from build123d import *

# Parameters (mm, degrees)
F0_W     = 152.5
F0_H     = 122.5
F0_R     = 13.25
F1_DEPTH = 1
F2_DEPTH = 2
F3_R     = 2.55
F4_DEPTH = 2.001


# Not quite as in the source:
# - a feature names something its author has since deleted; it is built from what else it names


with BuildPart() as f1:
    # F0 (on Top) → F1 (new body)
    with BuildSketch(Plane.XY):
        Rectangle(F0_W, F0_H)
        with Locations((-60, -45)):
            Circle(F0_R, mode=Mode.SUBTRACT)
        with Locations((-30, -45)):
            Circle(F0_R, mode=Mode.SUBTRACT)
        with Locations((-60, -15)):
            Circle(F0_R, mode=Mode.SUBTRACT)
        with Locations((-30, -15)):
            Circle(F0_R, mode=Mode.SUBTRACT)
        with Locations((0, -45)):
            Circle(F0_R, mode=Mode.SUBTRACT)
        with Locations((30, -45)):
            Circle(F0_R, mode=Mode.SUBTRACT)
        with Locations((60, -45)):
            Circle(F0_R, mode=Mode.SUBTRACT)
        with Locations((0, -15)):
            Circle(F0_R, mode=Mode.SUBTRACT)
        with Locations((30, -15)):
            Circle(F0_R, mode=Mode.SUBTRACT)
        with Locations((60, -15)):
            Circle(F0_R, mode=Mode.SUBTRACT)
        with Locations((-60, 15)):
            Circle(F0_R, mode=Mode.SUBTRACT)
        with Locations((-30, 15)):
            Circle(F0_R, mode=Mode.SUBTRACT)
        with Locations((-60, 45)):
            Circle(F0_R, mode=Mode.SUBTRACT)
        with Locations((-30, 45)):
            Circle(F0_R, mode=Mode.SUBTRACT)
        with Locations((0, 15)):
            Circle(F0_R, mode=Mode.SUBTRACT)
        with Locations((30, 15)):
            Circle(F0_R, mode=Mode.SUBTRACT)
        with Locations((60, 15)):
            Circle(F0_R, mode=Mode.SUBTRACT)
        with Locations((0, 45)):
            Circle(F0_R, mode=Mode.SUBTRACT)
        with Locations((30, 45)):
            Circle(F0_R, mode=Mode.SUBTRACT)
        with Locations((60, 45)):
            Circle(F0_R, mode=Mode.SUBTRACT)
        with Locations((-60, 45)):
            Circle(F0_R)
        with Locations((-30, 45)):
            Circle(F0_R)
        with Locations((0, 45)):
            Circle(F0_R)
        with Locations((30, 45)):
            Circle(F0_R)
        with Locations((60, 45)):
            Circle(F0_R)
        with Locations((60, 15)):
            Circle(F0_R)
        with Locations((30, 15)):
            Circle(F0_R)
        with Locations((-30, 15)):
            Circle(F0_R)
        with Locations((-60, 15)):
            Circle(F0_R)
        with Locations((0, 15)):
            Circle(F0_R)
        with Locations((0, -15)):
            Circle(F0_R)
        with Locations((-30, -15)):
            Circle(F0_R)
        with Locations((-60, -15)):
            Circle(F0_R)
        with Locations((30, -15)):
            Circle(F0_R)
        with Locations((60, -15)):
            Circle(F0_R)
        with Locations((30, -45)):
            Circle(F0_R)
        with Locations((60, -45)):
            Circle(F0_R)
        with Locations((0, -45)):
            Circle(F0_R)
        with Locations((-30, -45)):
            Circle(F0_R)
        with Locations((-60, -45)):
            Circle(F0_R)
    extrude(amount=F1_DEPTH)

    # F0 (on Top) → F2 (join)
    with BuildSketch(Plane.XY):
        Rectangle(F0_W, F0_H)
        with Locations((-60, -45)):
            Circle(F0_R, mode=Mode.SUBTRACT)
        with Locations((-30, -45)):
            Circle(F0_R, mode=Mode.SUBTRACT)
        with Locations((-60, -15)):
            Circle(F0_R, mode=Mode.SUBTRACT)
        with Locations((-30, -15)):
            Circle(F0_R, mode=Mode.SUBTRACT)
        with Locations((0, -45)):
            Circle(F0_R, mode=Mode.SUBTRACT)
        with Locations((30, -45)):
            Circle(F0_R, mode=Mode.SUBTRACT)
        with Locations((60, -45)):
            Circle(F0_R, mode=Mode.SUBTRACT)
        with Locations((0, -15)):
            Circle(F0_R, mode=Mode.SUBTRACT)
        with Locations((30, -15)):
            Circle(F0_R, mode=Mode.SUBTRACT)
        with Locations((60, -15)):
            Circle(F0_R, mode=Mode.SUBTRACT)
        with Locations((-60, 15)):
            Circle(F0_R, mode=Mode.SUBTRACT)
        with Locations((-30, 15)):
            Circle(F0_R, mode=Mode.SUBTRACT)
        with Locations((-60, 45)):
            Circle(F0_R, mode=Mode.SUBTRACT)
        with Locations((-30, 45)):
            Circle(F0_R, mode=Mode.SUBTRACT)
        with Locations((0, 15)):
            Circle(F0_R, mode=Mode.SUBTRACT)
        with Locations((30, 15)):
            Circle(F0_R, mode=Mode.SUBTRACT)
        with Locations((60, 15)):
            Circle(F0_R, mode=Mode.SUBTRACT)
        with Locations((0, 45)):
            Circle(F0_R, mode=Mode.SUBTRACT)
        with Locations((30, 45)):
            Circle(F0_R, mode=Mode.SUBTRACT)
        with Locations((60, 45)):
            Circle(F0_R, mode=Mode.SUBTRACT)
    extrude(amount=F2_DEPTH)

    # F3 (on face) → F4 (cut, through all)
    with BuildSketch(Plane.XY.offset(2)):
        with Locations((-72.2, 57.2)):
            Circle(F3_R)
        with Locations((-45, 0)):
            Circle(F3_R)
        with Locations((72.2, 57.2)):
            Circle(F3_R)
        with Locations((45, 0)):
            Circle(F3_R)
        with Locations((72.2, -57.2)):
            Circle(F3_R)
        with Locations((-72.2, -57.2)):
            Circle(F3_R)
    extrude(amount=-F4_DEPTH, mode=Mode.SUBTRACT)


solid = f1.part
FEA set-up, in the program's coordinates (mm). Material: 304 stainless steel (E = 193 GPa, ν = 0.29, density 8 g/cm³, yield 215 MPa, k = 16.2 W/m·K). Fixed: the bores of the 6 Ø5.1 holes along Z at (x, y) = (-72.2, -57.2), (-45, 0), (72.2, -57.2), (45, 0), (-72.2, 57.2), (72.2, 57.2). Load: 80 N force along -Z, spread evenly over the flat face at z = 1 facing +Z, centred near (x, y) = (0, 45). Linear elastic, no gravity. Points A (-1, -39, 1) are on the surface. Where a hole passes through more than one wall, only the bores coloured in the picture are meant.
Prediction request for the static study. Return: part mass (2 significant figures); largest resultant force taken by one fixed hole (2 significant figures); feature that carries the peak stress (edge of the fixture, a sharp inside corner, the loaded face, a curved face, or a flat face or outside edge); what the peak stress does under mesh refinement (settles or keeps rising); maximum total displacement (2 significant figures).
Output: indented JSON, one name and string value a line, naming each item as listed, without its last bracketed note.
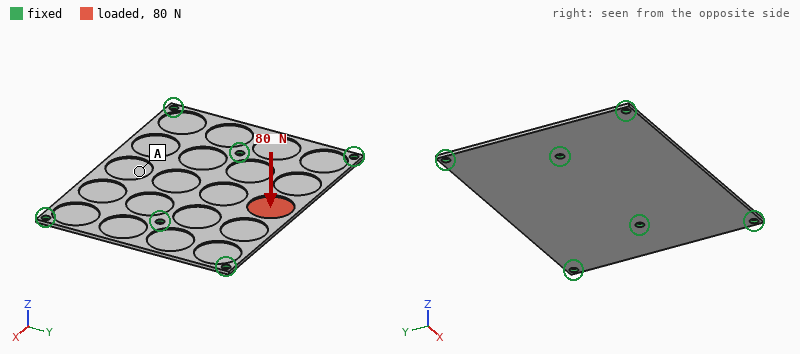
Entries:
{
  "part mass": "210 g",
  "largest resultant force taken by one fixed hole": "44 N",
  "feature that carries the peak stress": "a sharp inside corner",
  "what the peak stress does under mesh refinement": "keeps rising",
  "maximum total displacement": "0.37 mm"
}
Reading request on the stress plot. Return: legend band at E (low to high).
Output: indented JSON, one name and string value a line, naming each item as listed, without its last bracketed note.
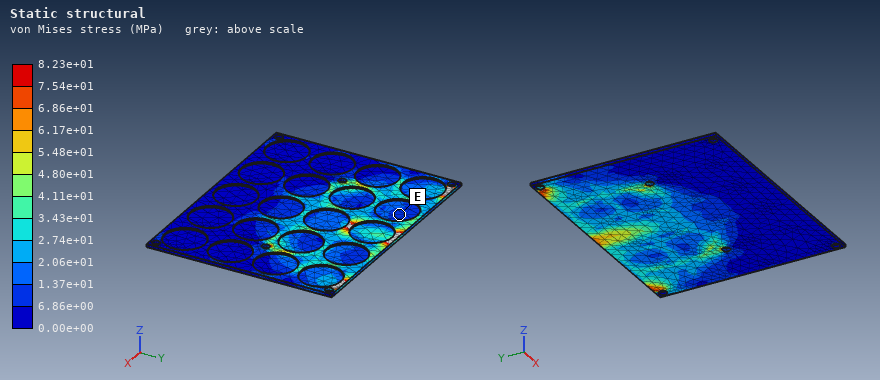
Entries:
{
  "legend band at E": "6.86e+00 to 1.37e+01 MPa"
}
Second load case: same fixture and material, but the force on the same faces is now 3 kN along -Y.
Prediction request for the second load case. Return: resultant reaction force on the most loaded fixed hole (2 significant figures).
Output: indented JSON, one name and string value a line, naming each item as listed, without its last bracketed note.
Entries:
{
  "resultant reaction force on the most loaded fixed hole": "1.2 kN"
}
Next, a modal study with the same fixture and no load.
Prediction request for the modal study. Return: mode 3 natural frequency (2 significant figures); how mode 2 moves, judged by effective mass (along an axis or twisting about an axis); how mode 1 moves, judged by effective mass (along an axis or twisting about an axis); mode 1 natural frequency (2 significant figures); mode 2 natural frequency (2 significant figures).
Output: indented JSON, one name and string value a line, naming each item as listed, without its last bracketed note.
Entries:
{
  "mode 3 natural frequency": "1200 Hz",
  "how mode 2 moves, judged by effective mass": "along Z",
  "how mode 1 moves, judged by effective mass": "twisting about X",
  "mode 1 natural frequency": "530 Hz",
  "mode 2 natural frequency": "560 Hz"
}
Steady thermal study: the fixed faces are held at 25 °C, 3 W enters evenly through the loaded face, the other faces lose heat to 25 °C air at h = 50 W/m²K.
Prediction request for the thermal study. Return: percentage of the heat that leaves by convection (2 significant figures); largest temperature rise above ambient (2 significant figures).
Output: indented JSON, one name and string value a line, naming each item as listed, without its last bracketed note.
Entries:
{
  "percentage of the heat that leaves by convection": "98 %",
  "largest temperature rise above ambient": "27 K"
}
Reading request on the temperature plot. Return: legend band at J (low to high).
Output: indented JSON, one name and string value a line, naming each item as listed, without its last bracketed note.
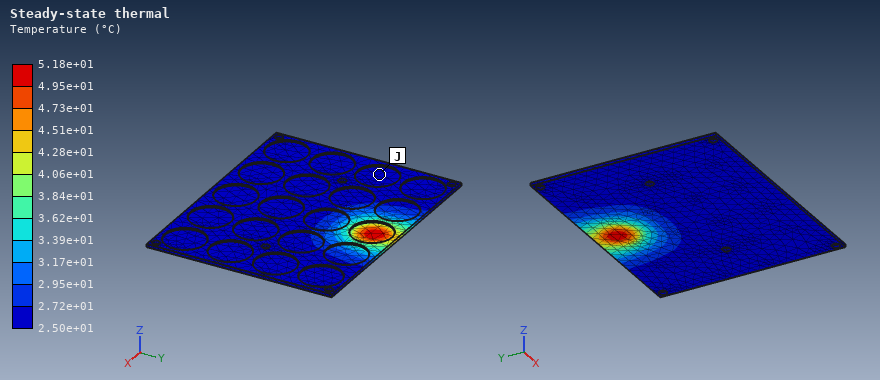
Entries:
{
  "legend band at J": "2.50e+01 to 2.72e+01 °C"
}
